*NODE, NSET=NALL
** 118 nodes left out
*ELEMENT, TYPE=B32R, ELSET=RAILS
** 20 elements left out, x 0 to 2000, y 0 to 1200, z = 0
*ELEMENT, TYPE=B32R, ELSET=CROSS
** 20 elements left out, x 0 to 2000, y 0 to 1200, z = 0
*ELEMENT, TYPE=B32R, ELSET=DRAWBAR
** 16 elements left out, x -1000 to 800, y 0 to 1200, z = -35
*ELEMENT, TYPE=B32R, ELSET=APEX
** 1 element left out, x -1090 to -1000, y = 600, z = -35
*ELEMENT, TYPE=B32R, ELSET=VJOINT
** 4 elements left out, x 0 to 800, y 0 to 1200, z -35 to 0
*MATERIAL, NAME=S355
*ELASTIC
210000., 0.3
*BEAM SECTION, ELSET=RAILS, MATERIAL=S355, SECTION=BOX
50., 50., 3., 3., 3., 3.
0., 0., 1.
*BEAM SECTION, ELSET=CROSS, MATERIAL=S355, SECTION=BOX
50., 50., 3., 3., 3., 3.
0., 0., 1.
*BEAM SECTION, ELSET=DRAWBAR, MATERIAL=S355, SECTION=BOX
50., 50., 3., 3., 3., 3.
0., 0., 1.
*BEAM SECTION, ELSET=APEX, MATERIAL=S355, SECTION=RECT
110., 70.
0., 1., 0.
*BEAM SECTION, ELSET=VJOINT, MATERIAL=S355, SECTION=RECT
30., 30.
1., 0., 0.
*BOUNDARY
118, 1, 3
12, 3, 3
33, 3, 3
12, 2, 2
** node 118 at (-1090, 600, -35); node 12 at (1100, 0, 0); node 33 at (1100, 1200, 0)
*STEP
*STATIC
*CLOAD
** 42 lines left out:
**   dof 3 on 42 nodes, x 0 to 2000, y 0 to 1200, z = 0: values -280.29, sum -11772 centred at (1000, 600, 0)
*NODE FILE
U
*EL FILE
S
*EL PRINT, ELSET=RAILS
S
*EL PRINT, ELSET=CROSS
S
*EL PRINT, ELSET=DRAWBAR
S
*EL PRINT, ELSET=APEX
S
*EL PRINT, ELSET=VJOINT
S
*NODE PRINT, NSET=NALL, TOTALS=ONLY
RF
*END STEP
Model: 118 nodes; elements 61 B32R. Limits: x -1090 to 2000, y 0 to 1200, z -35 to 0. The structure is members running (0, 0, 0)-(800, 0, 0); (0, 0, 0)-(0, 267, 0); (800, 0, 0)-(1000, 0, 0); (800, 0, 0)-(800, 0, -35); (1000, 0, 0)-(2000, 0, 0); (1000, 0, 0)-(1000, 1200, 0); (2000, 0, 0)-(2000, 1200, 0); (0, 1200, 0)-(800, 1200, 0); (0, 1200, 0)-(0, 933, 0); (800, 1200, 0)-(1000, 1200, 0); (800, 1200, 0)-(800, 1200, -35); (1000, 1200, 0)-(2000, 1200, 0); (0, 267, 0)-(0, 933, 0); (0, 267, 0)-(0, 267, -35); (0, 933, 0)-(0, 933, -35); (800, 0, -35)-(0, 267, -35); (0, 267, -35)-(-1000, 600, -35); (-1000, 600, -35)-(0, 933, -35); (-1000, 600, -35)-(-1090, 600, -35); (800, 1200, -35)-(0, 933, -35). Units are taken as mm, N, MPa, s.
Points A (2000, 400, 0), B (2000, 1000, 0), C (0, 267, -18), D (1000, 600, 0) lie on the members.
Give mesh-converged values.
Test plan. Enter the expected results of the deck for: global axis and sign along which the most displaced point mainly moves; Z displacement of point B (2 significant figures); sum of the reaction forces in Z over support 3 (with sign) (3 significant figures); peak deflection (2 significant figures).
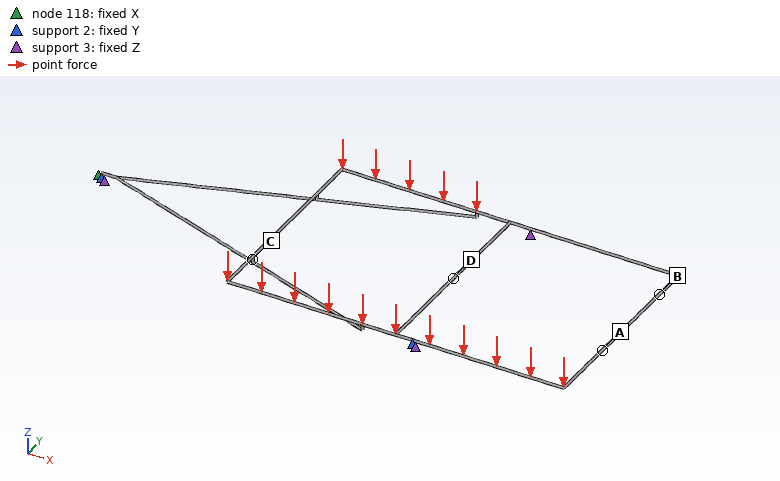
-Z
-9.7 mm
11800 N
9.7 mm
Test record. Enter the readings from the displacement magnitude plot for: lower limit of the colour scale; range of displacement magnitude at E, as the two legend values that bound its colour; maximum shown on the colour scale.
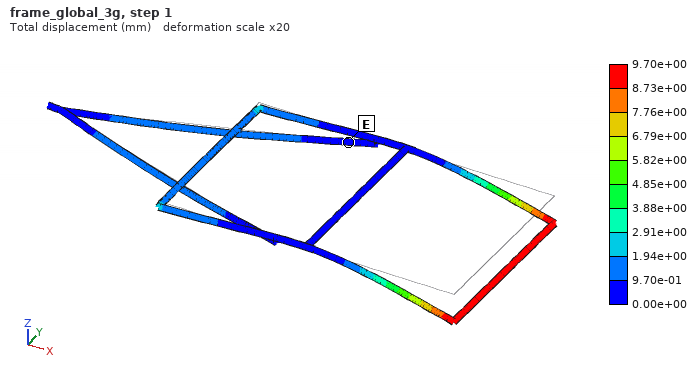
0.00e+00 mm
0.00e+00 to 9.70e-01 mm
9.70e+00 mm
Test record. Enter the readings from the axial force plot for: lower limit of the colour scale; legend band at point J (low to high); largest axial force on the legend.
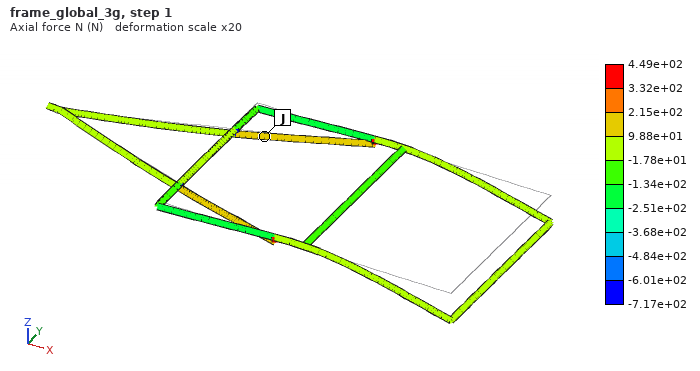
-7.17e+02 N
9.88e+01 to 2.15e+02 N
4.49e+02 N
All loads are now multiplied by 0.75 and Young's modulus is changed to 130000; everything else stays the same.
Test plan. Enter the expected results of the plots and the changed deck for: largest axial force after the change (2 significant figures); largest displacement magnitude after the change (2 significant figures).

340 N
12 mm
